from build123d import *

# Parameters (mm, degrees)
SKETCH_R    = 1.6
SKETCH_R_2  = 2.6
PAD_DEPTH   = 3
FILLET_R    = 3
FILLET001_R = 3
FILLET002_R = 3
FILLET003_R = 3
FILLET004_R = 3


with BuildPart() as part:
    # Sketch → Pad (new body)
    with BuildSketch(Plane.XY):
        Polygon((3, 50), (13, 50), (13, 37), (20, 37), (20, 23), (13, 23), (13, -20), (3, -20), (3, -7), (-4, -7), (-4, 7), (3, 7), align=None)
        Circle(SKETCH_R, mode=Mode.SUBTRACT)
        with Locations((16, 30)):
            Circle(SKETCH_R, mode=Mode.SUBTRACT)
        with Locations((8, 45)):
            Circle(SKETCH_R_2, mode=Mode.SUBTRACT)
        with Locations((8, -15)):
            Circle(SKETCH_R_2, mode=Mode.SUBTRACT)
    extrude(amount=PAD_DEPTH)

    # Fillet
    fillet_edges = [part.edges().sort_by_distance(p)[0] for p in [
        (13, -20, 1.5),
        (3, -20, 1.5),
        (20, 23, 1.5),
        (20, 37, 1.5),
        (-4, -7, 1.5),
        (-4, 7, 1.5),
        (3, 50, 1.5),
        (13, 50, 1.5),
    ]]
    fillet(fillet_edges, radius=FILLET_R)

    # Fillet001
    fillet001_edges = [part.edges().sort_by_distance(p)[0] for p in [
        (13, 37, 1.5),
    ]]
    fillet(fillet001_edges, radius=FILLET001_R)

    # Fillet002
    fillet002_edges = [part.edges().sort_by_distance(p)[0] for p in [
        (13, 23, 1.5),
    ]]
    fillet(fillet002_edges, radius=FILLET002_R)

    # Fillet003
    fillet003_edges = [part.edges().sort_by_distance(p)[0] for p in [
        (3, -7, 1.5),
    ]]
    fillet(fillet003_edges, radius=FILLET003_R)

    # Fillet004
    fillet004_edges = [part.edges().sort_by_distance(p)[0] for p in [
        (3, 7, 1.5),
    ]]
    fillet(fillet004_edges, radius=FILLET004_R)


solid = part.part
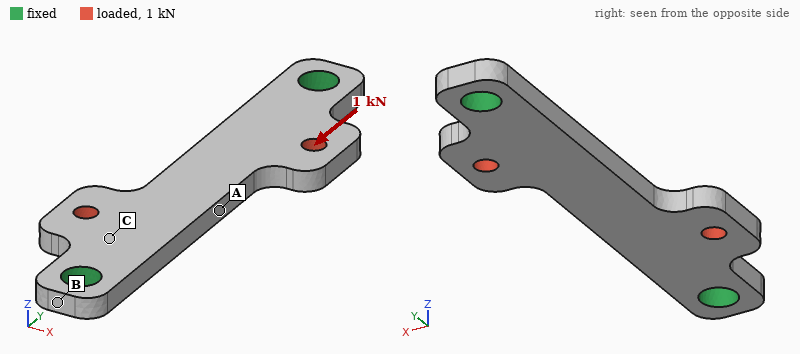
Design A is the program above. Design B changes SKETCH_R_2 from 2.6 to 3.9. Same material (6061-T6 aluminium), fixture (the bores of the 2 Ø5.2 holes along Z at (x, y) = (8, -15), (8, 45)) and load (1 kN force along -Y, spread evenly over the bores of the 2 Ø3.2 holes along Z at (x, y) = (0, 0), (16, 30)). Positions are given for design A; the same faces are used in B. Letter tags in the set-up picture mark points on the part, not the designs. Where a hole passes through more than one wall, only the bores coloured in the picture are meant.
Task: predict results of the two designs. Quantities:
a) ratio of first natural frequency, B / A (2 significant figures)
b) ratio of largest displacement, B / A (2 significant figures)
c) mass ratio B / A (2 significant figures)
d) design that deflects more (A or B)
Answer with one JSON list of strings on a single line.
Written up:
["1.1", "0.84", "0.94", "A"]
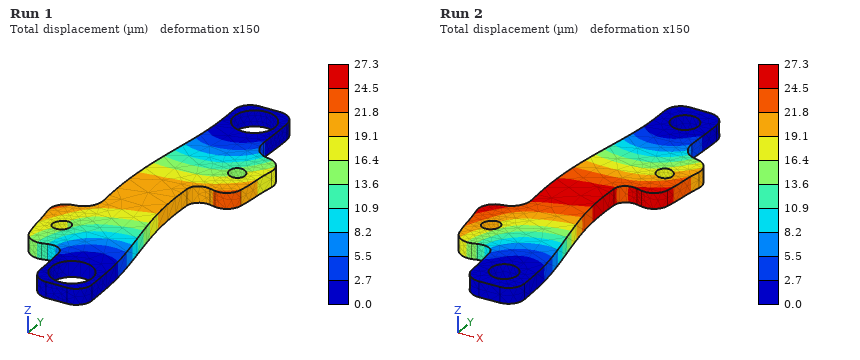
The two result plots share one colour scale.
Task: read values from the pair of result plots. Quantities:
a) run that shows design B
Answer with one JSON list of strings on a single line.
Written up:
["Run 1"]
